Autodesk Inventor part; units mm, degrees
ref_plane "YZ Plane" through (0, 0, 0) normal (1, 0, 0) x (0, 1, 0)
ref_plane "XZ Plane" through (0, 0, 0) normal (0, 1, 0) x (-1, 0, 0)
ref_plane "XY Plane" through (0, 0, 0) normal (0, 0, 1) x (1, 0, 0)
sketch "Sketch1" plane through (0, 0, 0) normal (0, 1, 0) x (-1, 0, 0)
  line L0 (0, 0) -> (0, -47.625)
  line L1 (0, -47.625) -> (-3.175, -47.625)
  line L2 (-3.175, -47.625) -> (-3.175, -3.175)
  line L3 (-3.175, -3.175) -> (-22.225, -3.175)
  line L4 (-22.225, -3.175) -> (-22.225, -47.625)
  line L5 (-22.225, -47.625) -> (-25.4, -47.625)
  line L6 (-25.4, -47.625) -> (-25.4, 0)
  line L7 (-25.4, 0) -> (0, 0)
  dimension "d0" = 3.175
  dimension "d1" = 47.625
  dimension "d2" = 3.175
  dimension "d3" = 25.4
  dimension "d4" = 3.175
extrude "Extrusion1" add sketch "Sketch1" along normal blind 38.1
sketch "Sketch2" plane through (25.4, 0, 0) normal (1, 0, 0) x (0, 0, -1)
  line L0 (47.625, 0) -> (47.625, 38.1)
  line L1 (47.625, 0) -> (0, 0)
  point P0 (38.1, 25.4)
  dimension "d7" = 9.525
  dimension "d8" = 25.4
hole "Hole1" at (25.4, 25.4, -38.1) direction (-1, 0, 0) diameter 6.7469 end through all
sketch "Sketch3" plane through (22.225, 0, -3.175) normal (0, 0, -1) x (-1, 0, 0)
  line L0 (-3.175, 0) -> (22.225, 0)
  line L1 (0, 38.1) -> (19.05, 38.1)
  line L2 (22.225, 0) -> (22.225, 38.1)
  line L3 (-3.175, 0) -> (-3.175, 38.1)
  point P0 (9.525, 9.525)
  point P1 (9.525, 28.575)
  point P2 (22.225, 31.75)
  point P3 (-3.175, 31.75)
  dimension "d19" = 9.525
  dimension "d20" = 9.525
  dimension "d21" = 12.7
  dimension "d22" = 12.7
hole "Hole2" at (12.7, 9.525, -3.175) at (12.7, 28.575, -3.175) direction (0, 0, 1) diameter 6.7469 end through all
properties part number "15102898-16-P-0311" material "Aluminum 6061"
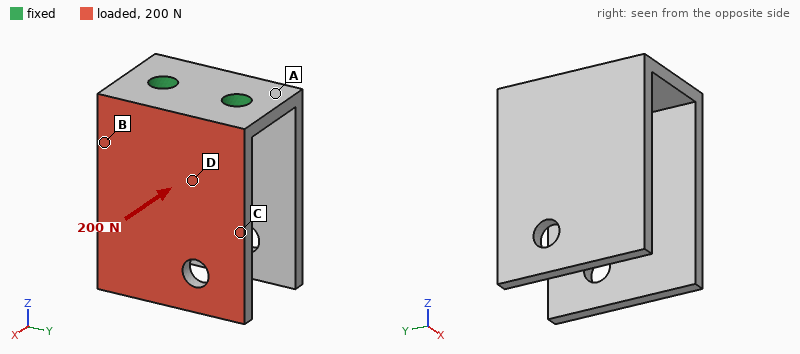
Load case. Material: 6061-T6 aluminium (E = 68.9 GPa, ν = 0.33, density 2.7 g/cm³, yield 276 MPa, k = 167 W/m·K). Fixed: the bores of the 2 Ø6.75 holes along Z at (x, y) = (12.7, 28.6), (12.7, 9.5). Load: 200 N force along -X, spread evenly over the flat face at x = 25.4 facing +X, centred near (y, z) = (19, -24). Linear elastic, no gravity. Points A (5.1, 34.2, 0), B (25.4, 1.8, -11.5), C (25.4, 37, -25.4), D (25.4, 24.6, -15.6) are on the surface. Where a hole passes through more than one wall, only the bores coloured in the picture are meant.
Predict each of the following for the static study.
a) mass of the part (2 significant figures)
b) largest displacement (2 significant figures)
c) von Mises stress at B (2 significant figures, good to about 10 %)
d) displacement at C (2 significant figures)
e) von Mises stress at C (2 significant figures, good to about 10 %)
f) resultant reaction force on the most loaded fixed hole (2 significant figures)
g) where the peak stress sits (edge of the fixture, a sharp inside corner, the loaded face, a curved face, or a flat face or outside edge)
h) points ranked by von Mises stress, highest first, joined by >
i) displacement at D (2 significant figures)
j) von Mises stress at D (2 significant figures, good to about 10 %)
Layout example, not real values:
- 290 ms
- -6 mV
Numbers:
- 36 g
- 0.53 mm
- 43 MPa
- 0.23 mm
- 16 MPa
- 110 N
- a flat face or outside edge
- B > D > C > A
- 0.12 mm
- 29 MPa
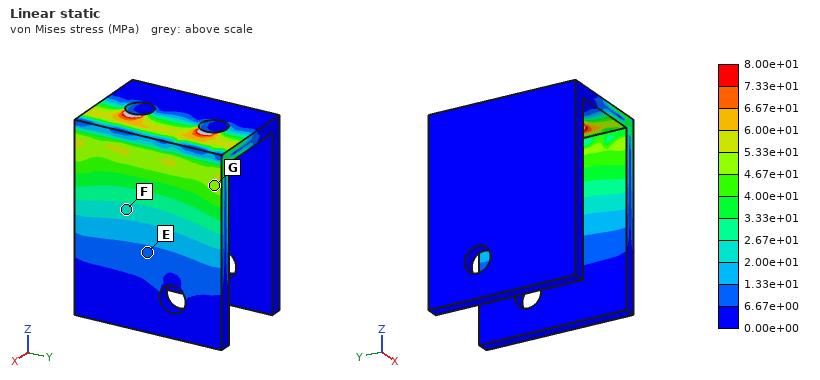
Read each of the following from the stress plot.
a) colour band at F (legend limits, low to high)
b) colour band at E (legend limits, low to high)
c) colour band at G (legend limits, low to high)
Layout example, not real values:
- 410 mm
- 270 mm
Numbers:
- 2.00e+01 to 2.67e+01 MPa
- 6.67e+00 to 1.33e+01 MPa
- 4.67e+01 to 5.33e+01 MPa
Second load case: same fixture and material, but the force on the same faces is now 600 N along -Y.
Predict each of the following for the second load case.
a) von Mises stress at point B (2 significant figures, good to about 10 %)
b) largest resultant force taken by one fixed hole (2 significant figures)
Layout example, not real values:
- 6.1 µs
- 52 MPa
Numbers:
- 12 MPa
- 680 N
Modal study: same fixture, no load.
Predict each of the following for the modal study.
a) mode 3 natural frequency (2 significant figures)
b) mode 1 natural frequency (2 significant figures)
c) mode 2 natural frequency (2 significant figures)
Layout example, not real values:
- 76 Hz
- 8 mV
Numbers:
- 2700 Hz
- 990 Hz
- 990 Hz
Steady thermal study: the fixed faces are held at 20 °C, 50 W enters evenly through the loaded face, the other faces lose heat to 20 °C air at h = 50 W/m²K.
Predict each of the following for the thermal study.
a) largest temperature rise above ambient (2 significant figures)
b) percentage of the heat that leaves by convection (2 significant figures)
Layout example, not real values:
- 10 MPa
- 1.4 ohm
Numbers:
- 66 K
- 13 %
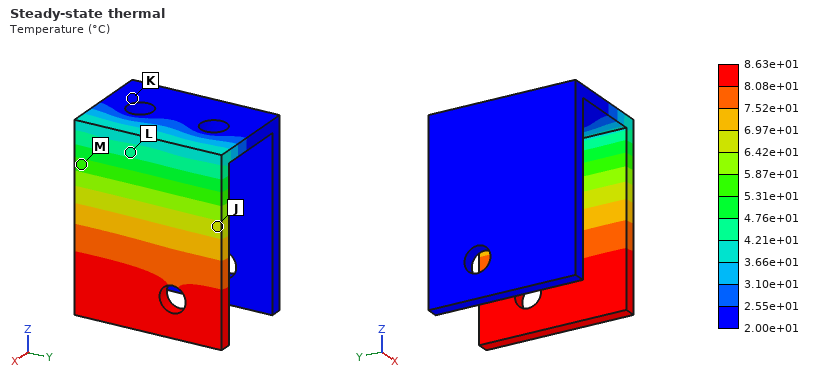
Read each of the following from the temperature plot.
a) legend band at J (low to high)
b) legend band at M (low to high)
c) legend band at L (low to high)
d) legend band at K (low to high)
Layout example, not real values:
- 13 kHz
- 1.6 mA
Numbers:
- 6.42e+01 to 6.97e+01 °C
- 5.31e+01 to 5.87e+01 °C
- 4.21e+01 to 4.76e+01 °C
- 2.00e+01 to 2.55e+01 °C
